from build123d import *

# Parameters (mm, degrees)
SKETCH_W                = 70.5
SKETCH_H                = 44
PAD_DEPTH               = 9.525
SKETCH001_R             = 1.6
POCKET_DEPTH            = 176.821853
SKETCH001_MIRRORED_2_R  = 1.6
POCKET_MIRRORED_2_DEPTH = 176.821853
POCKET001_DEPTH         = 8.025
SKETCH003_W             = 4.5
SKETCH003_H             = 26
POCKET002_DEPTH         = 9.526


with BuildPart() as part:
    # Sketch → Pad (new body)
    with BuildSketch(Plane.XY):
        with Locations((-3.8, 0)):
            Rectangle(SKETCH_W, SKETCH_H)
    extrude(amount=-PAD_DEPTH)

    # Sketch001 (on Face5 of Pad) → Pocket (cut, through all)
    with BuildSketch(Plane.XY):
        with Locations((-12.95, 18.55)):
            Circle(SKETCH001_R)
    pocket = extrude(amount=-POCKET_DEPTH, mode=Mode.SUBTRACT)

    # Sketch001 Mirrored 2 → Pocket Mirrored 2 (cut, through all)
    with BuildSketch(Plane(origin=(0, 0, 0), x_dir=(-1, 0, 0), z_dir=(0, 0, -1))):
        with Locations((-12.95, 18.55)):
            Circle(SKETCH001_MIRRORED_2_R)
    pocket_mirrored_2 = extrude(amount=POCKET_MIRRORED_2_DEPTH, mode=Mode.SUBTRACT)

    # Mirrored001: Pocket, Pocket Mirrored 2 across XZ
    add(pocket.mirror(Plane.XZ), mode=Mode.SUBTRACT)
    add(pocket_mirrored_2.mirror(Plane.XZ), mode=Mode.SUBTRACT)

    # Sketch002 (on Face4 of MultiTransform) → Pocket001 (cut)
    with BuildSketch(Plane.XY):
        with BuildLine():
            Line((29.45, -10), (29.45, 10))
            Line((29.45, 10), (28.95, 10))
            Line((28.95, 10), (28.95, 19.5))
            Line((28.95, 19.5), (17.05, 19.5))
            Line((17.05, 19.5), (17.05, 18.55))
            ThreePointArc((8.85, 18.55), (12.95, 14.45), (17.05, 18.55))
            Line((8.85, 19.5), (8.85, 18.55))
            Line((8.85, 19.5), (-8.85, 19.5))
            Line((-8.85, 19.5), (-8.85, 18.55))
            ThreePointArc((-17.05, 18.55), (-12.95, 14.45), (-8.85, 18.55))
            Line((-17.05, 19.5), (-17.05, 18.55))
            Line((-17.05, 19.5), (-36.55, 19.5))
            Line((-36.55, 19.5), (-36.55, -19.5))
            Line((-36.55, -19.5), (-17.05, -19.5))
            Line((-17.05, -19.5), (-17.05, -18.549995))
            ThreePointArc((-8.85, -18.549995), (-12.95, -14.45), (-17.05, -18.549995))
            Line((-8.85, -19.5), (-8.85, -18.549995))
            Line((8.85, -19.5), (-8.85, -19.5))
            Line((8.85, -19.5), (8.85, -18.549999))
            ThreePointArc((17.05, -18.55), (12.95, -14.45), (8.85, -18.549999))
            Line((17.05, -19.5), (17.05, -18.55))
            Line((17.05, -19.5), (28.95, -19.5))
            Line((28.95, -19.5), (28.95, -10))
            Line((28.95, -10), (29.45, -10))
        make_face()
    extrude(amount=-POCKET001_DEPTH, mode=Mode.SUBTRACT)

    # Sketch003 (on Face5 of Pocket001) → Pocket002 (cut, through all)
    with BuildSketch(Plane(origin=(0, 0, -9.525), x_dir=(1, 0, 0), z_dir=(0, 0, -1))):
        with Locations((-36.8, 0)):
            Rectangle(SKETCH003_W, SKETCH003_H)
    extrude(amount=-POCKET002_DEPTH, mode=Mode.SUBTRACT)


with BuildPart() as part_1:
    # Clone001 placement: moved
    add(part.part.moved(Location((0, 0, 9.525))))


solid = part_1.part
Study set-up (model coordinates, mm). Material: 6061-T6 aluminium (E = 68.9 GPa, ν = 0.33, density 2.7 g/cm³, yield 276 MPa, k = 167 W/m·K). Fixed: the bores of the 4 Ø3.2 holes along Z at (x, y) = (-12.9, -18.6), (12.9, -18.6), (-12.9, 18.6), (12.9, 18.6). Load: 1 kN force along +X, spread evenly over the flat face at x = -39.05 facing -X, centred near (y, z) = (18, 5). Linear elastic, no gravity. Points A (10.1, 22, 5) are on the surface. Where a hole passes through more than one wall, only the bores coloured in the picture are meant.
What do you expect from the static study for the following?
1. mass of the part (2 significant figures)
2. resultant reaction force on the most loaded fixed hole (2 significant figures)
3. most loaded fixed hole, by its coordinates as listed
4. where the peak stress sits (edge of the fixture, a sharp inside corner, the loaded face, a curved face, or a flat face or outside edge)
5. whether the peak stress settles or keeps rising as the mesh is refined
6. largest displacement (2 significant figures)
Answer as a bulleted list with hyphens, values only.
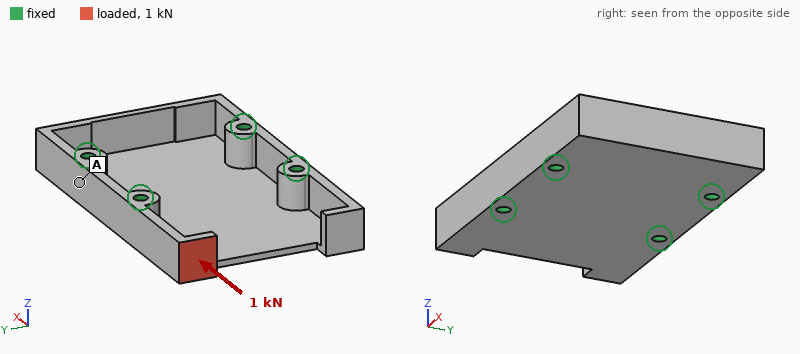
- 24 g
- 880 N
- (-12.9, 18.6)
- a sharp inside corner
- keeps rising
- 94 µm
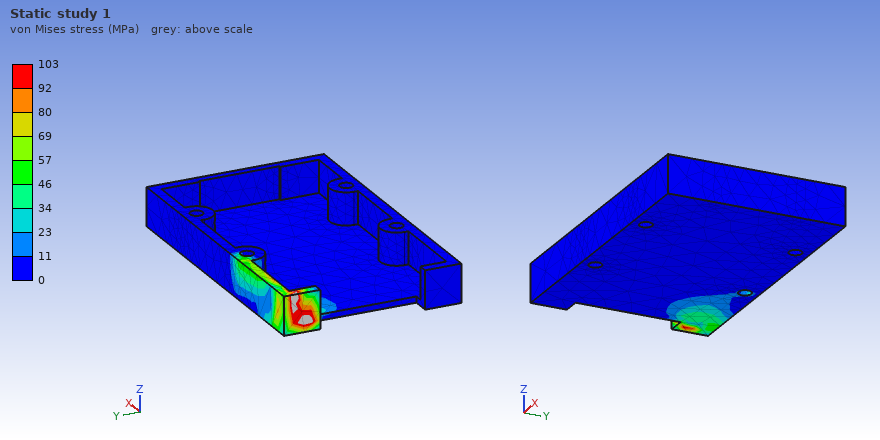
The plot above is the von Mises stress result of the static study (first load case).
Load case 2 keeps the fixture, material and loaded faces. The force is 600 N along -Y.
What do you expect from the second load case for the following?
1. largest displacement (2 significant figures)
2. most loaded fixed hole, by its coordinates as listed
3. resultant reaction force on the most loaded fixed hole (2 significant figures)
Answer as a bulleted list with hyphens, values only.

- 0.28 mm
- (-12.9, 18.6)
- 500 N
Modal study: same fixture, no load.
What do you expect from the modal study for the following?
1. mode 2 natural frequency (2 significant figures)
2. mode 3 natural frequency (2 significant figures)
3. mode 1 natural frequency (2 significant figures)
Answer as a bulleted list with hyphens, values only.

- 7300 Hz
- 7600 Hz
- 4900 Hz
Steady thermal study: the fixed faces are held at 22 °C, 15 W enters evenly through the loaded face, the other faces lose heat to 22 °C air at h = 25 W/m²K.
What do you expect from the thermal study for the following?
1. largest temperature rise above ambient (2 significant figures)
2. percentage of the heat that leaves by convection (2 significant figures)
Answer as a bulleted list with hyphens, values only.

- 55 K
- 6.4 %
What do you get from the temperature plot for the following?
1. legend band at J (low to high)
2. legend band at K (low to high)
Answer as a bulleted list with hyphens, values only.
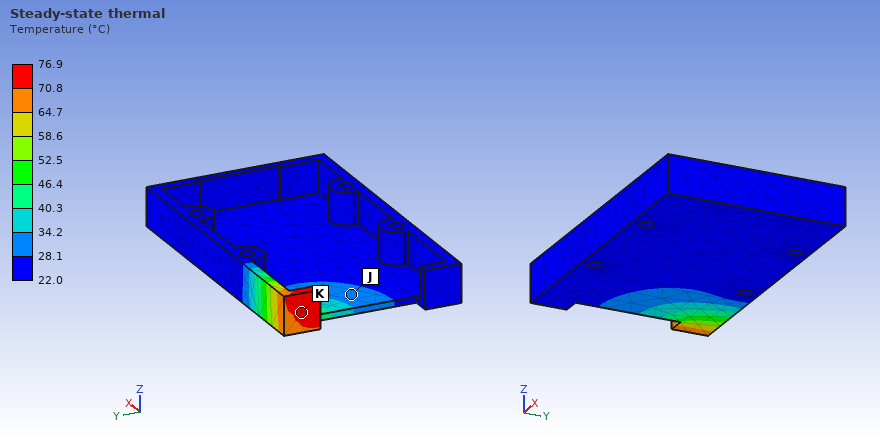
- 28.1 to 34.2 °C
- 70.8 to 76.9 °C
